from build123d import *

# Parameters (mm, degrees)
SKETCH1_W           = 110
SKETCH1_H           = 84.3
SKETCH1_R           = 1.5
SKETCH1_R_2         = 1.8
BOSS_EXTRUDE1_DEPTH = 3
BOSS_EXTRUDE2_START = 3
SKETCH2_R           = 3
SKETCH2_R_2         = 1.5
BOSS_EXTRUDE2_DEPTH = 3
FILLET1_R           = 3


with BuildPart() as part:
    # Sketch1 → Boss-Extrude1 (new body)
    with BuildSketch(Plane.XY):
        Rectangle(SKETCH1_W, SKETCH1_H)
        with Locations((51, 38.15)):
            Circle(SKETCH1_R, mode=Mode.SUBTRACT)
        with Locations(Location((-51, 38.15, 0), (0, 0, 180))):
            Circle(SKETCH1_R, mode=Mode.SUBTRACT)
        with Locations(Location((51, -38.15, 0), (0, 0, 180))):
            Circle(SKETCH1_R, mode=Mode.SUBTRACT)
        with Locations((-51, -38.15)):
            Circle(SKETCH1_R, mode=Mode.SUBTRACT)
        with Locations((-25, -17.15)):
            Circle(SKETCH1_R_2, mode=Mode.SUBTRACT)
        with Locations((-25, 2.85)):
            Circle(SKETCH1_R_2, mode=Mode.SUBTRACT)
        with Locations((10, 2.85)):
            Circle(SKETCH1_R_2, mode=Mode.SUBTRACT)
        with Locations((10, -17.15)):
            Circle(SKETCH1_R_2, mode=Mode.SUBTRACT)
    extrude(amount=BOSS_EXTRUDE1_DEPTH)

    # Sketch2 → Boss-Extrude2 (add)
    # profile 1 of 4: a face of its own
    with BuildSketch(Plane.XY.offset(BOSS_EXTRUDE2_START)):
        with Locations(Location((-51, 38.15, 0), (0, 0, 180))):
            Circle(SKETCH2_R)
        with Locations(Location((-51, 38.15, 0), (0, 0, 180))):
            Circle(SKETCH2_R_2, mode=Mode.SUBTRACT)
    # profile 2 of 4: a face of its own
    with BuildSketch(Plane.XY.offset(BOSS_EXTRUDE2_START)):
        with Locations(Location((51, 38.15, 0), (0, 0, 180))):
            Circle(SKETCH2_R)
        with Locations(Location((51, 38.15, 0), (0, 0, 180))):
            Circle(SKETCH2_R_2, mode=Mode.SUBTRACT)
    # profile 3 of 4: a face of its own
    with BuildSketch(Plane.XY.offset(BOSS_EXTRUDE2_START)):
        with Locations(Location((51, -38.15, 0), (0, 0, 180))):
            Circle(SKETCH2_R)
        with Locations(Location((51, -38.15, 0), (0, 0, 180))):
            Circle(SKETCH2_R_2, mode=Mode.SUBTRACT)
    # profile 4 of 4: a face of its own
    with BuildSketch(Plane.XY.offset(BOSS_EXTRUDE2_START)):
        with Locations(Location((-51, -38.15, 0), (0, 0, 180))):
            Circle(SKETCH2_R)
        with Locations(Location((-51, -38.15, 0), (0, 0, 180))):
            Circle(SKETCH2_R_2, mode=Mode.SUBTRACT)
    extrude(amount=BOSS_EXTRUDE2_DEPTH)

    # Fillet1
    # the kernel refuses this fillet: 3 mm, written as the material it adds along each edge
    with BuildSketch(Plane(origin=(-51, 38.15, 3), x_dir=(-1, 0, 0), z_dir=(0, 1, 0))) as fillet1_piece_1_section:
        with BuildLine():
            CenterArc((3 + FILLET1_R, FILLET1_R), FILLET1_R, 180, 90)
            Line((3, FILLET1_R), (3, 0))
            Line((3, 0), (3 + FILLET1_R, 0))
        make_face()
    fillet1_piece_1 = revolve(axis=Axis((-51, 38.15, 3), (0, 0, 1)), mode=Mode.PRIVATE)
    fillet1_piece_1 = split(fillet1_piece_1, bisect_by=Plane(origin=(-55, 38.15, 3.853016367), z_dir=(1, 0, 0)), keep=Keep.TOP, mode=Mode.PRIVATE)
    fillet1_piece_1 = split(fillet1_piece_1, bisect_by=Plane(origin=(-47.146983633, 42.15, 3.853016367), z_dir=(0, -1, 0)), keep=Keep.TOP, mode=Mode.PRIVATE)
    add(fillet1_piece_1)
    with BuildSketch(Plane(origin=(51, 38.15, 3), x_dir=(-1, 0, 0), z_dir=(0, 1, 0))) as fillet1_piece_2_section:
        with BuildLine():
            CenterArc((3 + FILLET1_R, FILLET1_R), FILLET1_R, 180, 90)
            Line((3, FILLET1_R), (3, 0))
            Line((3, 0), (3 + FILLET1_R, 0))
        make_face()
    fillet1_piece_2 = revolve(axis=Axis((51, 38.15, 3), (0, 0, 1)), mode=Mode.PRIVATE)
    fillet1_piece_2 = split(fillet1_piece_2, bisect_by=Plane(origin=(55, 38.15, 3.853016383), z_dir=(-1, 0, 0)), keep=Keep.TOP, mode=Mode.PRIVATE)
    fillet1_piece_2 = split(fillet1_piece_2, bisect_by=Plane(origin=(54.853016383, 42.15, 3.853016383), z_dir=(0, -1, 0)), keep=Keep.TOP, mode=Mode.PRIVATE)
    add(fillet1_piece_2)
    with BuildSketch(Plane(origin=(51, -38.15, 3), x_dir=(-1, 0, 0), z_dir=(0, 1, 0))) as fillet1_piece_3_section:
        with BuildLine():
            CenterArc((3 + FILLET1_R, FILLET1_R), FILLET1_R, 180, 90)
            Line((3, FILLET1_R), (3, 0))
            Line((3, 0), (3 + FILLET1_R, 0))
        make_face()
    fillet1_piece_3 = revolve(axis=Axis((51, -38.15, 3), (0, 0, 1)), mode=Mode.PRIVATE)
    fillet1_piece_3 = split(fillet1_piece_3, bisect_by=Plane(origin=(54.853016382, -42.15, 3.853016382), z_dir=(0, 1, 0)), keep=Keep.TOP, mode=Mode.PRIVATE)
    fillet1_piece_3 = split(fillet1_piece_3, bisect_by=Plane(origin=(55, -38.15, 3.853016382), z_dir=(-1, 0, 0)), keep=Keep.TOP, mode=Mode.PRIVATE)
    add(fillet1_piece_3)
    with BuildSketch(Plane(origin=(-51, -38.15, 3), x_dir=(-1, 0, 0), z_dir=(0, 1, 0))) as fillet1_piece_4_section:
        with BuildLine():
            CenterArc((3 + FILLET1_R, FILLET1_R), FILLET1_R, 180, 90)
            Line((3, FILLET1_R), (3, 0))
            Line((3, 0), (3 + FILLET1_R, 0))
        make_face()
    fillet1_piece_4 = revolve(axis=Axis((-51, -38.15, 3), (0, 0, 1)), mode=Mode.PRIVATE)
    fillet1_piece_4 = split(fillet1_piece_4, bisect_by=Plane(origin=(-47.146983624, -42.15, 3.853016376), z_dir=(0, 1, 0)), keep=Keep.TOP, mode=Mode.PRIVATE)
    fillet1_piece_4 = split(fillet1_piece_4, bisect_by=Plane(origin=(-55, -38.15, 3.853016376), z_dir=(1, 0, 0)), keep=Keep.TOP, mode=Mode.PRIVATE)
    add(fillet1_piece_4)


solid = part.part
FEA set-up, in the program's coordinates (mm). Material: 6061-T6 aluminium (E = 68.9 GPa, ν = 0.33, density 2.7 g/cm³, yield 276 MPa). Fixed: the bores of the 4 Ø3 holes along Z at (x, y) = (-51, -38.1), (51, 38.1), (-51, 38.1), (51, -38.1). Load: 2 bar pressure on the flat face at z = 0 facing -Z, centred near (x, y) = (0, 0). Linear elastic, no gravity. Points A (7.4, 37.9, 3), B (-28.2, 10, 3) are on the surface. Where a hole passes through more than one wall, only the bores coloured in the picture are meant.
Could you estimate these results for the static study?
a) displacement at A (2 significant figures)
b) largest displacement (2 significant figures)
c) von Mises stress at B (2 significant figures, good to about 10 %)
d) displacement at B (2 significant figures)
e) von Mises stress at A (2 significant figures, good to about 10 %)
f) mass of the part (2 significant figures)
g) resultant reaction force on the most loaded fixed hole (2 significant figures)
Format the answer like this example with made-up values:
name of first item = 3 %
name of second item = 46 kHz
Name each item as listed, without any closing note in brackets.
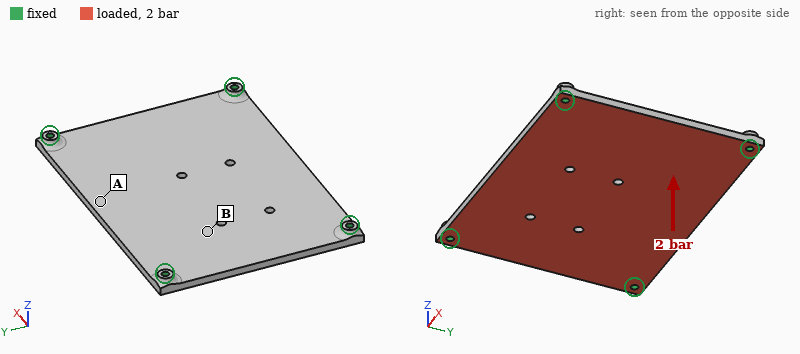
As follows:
displacement at A = 0.48 mm
largest displacement = 0.61 mm
von Mises stress at B = 36 MPa
displacement at B = 0.41 mm
von Mises stress at A = 72 MPa
mass of the part = 76 g
resultant reaction force on the most loaded fixed hole = 540 N
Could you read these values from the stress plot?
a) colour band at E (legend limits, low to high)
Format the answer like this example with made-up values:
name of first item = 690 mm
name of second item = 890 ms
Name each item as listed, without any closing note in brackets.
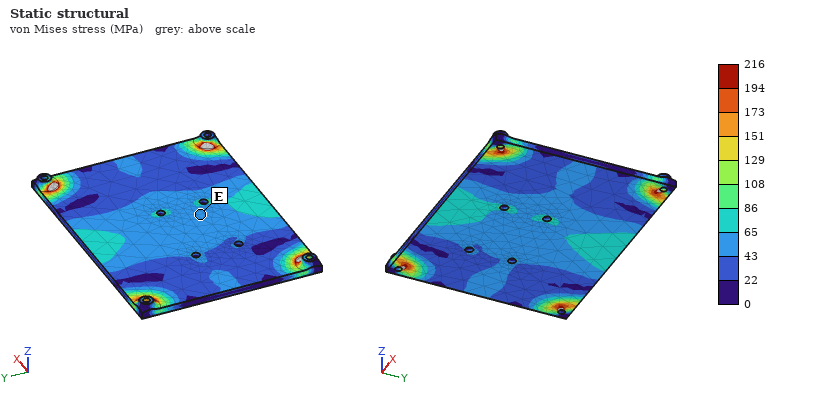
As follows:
colour band at E = 43 to 65 MPa
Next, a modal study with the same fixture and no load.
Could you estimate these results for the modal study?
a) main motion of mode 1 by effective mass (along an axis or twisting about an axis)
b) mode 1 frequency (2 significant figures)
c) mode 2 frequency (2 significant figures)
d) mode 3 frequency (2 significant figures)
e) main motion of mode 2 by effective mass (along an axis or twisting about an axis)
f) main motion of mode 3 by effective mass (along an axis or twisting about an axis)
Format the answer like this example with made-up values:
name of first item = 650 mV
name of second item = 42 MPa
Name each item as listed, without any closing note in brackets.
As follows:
main motion of mode 1 by effective mass = along Z
mode 1 frequency = 1200 Hz
mode 2 frequency = 2000 Hz
mode 3 frequency = 2700 Hz
main motion of mode 2 by effective mass = twisting about X
main motion of mode 3 by effective mass = twisting about Y
